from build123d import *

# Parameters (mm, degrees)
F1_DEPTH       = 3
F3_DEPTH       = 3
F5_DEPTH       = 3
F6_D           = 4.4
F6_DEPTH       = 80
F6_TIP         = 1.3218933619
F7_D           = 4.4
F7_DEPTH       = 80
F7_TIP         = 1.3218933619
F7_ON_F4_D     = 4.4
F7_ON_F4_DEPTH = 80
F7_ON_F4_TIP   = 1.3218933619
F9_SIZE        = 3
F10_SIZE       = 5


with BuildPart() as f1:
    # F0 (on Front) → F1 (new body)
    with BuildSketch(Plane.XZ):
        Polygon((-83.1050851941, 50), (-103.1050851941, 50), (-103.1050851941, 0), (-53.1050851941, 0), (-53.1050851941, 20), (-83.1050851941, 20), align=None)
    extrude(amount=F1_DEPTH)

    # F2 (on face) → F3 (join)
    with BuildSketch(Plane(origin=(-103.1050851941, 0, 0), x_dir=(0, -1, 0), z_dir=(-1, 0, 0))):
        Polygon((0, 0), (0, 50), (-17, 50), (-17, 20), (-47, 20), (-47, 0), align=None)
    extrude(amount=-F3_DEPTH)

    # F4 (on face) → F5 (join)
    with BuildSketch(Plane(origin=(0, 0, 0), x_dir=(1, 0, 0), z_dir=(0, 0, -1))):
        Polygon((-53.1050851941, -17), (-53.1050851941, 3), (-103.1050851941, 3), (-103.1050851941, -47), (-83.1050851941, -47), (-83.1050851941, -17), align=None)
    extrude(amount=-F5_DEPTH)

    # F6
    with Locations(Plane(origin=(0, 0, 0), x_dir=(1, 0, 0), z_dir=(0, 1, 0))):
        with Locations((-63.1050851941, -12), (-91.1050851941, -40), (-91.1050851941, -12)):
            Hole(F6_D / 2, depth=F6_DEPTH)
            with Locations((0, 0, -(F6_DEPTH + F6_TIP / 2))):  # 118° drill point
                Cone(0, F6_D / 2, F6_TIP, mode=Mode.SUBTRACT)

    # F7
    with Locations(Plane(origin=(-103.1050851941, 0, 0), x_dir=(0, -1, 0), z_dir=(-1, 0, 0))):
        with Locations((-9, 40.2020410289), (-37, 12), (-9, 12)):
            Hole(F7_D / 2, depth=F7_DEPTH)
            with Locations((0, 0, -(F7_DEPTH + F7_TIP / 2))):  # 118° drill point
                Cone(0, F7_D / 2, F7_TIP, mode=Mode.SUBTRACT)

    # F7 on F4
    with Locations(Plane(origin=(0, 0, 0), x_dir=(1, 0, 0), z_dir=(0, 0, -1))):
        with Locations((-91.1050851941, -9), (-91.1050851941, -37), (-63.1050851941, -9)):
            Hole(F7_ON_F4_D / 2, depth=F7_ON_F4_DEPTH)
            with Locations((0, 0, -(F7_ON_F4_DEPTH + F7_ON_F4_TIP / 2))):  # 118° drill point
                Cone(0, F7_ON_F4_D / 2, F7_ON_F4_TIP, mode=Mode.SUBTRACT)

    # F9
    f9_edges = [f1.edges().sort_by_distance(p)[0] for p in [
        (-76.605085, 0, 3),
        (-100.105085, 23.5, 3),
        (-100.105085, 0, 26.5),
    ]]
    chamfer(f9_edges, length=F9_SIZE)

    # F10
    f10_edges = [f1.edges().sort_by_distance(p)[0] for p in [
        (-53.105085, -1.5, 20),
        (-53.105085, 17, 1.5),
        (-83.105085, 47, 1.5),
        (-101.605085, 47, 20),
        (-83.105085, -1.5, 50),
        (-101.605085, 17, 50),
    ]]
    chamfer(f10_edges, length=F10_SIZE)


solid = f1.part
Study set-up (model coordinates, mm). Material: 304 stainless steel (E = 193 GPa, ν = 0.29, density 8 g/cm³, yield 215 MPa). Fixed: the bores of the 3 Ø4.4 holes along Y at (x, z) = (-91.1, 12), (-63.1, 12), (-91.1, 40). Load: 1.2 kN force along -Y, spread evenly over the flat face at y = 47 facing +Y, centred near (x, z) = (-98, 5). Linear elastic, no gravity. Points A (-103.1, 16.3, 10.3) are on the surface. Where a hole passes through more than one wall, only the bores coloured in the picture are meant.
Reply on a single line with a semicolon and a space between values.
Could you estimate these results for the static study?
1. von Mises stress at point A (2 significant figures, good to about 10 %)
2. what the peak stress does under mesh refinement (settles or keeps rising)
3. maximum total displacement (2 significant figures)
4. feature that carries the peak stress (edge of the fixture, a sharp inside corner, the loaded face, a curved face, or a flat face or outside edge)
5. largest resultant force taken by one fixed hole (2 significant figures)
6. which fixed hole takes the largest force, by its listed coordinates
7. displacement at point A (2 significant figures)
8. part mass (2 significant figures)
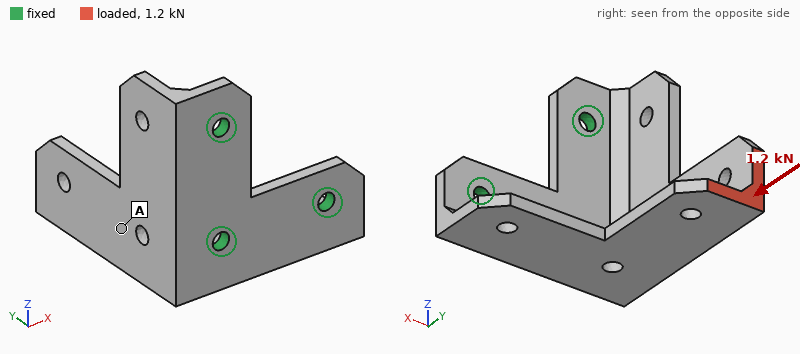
16 MPa; keeps rising; 49 µm; edge of the fixture; 1.6 kN; (-91.1, 12); 21 µm; 100 g
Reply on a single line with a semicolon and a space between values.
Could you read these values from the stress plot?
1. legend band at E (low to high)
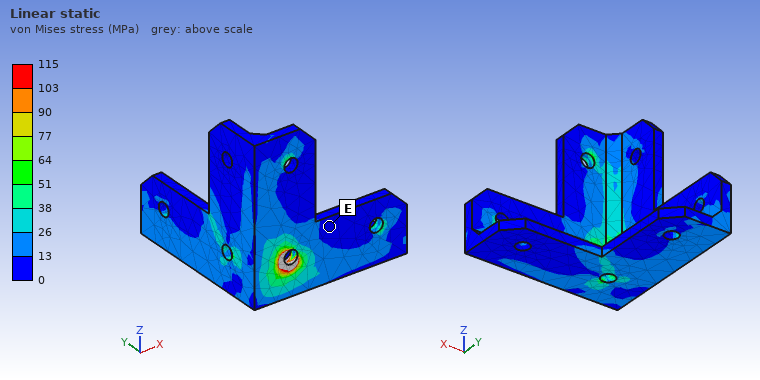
0 to 13 MPa
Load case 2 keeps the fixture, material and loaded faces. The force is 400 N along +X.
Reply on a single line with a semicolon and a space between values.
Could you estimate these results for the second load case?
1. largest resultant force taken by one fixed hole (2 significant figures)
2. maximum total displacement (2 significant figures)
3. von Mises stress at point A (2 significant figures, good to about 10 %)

720 N; 87 µm; 23 MPa
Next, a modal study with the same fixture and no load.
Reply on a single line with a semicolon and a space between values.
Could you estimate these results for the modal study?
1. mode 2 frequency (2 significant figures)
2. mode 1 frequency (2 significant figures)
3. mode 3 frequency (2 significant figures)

3100 Hz; 3000 Hz; 6100 Hz
